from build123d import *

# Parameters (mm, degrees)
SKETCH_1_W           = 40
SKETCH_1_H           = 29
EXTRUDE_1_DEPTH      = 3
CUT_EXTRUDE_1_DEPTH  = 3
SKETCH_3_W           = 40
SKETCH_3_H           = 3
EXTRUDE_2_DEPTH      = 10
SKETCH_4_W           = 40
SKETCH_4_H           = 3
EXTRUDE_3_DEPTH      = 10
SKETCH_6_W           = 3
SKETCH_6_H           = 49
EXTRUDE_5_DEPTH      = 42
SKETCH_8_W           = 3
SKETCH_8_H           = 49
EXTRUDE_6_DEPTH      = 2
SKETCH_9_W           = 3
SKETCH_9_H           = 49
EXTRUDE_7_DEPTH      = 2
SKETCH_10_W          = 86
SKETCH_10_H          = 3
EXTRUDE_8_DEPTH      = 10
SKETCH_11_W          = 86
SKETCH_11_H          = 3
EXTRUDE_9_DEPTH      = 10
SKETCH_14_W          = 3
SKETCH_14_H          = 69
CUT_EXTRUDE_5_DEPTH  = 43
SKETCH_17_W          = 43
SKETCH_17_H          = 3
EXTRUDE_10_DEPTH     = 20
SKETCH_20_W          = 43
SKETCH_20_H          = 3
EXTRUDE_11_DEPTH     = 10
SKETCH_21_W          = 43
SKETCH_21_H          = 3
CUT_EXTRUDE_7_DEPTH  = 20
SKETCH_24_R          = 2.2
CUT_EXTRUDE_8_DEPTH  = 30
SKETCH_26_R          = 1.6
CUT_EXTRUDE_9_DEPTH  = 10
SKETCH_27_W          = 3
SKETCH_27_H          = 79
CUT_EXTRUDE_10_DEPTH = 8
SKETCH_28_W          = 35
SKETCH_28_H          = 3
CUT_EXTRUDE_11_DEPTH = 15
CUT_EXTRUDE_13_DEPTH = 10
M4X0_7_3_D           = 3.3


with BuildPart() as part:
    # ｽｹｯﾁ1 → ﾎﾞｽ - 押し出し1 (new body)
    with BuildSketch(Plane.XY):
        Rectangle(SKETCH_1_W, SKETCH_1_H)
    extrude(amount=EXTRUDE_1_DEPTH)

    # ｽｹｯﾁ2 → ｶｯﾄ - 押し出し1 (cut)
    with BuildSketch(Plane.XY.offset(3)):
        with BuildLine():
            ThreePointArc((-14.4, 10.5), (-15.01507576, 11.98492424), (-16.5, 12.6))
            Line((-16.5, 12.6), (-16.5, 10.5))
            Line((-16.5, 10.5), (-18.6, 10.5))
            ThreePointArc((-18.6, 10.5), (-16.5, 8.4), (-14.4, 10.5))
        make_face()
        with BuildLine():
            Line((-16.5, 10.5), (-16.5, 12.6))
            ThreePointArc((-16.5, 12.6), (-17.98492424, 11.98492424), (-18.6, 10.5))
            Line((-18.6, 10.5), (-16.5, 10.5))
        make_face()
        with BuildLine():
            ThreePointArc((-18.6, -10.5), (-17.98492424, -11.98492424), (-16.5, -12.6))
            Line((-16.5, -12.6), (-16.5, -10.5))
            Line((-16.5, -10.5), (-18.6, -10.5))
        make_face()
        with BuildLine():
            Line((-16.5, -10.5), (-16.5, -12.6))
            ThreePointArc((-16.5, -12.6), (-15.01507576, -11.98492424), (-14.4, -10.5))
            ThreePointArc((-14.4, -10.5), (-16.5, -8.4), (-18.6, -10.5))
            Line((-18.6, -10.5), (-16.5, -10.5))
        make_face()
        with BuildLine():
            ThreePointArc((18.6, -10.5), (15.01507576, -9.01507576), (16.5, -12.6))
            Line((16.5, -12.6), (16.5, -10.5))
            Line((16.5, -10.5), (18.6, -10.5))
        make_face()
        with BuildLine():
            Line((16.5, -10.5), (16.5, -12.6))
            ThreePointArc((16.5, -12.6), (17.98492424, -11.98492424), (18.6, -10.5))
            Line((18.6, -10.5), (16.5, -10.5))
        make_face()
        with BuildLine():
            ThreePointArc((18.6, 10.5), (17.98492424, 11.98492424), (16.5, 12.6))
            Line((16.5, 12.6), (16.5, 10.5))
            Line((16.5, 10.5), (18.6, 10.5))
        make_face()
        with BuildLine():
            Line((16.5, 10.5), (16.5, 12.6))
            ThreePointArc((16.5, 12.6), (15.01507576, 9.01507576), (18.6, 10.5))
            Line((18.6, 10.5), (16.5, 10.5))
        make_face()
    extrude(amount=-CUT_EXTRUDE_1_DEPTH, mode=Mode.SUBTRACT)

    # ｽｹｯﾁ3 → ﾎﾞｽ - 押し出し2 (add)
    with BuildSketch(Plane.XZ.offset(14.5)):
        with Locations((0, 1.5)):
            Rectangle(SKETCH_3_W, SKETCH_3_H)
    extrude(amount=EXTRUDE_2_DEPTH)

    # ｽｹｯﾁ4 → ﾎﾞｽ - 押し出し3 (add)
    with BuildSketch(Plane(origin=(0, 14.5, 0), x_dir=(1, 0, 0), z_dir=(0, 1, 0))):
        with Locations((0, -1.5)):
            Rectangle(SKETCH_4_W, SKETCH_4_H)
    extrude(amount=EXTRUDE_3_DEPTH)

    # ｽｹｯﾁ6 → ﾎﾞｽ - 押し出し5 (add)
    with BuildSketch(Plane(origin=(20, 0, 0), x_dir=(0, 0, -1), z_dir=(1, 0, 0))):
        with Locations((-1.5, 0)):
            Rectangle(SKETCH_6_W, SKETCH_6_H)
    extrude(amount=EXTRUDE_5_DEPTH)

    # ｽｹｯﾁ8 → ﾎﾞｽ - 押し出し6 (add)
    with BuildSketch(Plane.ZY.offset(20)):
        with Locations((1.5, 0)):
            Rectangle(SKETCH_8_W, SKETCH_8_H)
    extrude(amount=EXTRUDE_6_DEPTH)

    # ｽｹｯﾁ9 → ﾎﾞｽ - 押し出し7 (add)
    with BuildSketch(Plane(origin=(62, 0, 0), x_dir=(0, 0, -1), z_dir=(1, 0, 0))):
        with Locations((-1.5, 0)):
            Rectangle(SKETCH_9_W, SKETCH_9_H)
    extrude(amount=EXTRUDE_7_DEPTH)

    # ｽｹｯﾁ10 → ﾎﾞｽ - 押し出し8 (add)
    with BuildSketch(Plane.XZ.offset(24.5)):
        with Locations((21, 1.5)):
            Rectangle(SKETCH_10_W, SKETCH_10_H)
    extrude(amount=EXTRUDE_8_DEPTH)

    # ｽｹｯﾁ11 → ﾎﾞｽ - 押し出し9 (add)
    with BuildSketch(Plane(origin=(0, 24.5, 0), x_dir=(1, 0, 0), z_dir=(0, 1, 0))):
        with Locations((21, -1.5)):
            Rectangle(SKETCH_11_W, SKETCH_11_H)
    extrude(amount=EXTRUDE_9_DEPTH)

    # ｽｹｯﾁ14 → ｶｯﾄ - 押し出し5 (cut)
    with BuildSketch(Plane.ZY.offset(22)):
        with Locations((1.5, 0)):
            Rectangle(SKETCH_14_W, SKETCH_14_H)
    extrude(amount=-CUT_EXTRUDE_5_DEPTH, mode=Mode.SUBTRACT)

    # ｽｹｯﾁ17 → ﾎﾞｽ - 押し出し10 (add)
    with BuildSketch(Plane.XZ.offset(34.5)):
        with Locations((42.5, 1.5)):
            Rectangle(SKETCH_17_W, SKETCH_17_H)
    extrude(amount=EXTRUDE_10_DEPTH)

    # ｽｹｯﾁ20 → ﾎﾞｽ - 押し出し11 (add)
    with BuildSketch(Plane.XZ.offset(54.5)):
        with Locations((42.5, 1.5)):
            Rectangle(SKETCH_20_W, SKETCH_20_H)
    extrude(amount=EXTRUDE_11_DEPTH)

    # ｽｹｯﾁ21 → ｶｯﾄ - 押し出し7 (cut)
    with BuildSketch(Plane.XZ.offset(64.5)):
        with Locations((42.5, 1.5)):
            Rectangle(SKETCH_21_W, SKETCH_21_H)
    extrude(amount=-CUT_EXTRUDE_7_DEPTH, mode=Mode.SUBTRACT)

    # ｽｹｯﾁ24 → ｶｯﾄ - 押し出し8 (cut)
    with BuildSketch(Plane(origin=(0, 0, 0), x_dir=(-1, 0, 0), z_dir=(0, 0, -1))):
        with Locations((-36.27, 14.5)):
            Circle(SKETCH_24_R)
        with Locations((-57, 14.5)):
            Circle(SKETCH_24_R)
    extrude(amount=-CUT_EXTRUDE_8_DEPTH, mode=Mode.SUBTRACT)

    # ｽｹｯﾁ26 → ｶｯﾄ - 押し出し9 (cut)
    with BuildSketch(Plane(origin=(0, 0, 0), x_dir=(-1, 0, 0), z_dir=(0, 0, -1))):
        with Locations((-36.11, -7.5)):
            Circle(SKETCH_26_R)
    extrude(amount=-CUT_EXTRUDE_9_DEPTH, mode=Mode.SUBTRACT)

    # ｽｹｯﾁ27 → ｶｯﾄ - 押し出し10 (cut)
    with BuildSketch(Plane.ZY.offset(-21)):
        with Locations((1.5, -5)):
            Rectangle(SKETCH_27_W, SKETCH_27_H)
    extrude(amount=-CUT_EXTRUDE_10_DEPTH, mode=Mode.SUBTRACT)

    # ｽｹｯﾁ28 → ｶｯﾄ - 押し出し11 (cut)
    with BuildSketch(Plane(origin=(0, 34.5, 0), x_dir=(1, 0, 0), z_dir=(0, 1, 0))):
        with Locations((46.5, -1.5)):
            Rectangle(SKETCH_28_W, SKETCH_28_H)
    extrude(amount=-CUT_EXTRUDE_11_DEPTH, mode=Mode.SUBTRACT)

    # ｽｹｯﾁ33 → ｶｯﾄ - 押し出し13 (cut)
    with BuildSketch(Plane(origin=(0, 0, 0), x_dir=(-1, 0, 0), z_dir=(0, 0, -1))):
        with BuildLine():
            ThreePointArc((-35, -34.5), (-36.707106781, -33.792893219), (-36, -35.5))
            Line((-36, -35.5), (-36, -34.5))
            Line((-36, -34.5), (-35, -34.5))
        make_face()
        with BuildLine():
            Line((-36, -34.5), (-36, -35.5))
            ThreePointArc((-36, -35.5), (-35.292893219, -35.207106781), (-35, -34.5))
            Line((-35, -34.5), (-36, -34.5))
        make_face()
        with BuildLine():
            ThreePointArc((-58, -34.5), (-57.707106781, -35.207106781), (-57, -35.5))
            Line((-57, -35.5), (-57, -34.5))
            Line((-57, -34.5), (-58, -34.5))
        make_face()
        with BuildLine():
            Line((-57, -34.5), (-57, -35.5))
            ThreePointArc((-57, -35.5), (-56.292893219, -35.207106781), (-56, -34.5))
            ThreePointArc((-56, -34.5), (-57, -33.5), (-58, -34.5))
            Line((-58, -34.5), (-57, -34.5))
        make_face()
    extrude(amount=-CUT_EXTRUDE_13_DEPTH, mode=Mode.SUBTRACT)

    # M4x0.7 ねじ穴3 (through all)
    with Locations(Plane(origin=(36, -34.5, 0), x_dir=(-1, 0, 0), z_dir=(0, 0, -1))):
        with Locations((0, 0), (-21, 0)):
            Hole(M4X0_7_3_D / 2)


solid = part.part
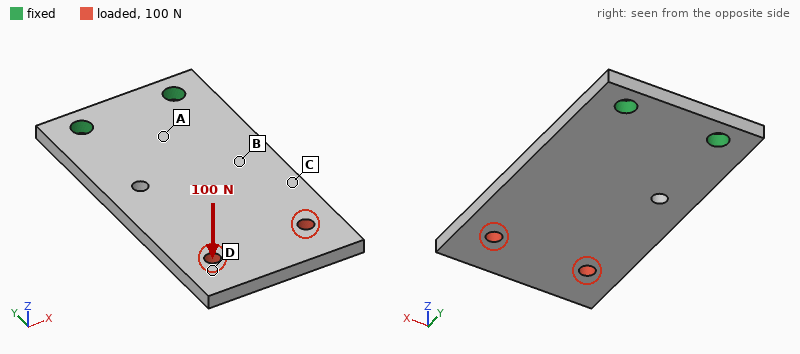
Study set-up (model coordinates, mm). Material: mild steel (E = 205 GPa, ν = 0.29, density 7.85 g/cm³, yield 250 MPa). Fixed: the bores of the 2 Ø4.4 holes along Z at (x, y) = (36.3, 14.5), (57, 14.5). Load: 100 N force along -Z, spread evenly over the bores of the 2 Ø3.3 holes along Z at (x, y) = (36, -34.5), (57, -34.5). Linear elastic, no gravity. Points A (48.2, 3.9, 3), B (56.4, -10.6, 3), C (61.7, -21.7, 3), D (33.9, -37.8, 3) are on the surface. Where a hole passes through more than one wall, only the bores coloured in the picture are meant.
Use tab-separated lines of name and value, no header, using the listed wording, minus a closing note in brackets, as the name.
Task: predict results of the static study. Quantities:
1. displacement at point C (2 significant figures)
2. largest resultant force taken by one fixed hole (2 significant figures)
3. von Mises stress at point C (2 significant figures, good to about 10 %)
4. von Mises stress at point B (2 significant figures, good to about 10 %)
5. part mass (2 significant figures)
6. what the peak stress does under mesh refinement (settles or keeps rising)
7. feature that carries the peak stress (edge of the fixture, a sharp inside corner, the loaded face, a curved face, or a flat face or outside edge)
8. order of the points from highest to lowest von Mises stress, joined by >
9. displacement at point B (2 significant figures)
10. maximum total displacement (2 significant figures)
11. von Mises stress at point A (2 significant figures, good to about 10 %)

displacement at point C	0.14 mm
largest resultant force taken by one fixed hole	51 N
von Mises stress at point C	26 MPa
von Mises stress at point B	45 MPa
part mass	51 g
what the peak stress does under mesh refinement	keeps rising
feature that carries the peak stress	edge of the fixture
order of the points from highest to lowest von Mises stress, joined by >	A > B > C > D
displacement at point B	0.074 mm
maximum total displacement	0.30 mm
von Mises stress at point A	67 MPa
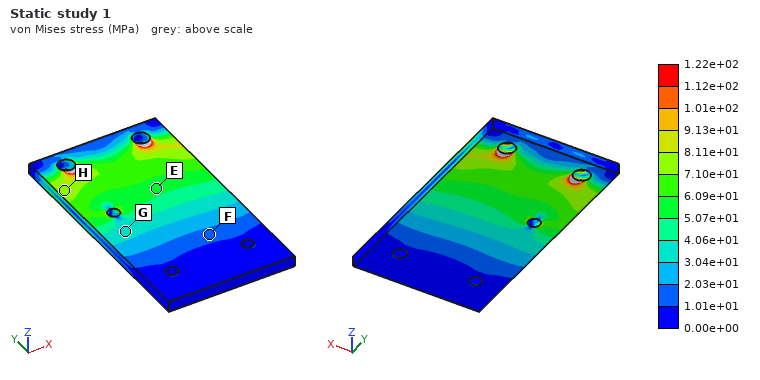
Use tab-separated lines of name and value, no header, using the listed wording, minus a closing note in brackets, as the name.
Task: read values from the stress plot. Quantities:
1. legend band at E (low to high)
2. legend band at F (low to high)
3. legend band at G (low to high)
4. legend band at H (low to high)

legend band at E	5.07e+01 to 6.09e+01 MPa
legend band at F	1.01e+01 to 2.03e+01 MPa
legend band at G	3.04e+01 to 4.06e+01 MPa
legend band at H	7.10e+01 to 8.11e+01 MPa
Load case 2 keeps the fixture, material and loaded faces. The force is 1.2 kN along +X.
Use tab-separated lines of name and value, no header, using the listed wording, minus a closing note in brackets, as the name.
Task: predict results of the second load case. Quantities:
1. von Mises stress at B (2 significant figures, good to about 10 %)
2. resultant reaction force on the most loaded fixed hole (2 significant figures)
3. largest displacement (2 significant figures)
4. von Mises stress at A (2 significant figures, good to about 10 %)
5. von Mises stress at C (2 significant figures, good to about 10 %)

von Mises stress at B	34 MPa
resultant reaction force on the most loaded fixed hole	2.6 kN
largest displacement	43 µm
von Mises stress at A	35 MPa
von Mises stress at C	23 MPa
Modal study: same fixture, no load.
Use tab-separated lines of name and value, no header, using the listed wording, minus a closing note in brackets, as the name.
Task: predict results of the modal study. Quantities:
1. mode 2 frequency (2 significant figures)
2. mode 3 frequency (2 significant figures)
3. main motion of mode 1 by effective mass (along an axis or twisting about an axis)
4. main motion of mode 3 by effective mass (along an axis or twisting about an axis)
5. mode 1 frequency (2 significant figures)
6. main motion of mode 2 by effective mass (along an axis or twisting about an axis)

mode 2 frequency	2700 Hz
mode 3 frequency	4500 Hz
main motion of mode 1 by effective mass	along Z
main motion of mode 3 by effective mass	along Z
mode 1 frequency	740 Hz
main motion of mode 2 by effective mass	twisting about Y
